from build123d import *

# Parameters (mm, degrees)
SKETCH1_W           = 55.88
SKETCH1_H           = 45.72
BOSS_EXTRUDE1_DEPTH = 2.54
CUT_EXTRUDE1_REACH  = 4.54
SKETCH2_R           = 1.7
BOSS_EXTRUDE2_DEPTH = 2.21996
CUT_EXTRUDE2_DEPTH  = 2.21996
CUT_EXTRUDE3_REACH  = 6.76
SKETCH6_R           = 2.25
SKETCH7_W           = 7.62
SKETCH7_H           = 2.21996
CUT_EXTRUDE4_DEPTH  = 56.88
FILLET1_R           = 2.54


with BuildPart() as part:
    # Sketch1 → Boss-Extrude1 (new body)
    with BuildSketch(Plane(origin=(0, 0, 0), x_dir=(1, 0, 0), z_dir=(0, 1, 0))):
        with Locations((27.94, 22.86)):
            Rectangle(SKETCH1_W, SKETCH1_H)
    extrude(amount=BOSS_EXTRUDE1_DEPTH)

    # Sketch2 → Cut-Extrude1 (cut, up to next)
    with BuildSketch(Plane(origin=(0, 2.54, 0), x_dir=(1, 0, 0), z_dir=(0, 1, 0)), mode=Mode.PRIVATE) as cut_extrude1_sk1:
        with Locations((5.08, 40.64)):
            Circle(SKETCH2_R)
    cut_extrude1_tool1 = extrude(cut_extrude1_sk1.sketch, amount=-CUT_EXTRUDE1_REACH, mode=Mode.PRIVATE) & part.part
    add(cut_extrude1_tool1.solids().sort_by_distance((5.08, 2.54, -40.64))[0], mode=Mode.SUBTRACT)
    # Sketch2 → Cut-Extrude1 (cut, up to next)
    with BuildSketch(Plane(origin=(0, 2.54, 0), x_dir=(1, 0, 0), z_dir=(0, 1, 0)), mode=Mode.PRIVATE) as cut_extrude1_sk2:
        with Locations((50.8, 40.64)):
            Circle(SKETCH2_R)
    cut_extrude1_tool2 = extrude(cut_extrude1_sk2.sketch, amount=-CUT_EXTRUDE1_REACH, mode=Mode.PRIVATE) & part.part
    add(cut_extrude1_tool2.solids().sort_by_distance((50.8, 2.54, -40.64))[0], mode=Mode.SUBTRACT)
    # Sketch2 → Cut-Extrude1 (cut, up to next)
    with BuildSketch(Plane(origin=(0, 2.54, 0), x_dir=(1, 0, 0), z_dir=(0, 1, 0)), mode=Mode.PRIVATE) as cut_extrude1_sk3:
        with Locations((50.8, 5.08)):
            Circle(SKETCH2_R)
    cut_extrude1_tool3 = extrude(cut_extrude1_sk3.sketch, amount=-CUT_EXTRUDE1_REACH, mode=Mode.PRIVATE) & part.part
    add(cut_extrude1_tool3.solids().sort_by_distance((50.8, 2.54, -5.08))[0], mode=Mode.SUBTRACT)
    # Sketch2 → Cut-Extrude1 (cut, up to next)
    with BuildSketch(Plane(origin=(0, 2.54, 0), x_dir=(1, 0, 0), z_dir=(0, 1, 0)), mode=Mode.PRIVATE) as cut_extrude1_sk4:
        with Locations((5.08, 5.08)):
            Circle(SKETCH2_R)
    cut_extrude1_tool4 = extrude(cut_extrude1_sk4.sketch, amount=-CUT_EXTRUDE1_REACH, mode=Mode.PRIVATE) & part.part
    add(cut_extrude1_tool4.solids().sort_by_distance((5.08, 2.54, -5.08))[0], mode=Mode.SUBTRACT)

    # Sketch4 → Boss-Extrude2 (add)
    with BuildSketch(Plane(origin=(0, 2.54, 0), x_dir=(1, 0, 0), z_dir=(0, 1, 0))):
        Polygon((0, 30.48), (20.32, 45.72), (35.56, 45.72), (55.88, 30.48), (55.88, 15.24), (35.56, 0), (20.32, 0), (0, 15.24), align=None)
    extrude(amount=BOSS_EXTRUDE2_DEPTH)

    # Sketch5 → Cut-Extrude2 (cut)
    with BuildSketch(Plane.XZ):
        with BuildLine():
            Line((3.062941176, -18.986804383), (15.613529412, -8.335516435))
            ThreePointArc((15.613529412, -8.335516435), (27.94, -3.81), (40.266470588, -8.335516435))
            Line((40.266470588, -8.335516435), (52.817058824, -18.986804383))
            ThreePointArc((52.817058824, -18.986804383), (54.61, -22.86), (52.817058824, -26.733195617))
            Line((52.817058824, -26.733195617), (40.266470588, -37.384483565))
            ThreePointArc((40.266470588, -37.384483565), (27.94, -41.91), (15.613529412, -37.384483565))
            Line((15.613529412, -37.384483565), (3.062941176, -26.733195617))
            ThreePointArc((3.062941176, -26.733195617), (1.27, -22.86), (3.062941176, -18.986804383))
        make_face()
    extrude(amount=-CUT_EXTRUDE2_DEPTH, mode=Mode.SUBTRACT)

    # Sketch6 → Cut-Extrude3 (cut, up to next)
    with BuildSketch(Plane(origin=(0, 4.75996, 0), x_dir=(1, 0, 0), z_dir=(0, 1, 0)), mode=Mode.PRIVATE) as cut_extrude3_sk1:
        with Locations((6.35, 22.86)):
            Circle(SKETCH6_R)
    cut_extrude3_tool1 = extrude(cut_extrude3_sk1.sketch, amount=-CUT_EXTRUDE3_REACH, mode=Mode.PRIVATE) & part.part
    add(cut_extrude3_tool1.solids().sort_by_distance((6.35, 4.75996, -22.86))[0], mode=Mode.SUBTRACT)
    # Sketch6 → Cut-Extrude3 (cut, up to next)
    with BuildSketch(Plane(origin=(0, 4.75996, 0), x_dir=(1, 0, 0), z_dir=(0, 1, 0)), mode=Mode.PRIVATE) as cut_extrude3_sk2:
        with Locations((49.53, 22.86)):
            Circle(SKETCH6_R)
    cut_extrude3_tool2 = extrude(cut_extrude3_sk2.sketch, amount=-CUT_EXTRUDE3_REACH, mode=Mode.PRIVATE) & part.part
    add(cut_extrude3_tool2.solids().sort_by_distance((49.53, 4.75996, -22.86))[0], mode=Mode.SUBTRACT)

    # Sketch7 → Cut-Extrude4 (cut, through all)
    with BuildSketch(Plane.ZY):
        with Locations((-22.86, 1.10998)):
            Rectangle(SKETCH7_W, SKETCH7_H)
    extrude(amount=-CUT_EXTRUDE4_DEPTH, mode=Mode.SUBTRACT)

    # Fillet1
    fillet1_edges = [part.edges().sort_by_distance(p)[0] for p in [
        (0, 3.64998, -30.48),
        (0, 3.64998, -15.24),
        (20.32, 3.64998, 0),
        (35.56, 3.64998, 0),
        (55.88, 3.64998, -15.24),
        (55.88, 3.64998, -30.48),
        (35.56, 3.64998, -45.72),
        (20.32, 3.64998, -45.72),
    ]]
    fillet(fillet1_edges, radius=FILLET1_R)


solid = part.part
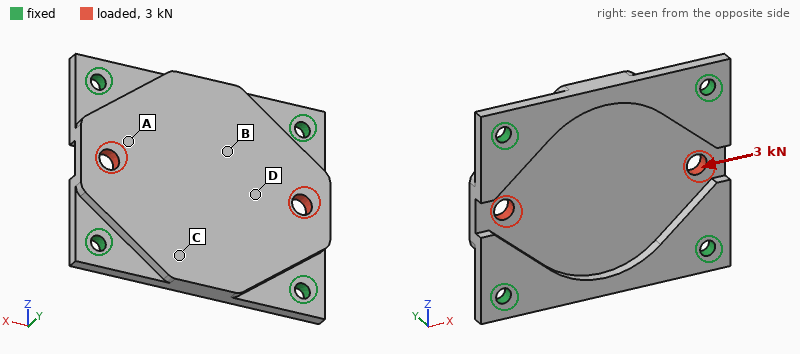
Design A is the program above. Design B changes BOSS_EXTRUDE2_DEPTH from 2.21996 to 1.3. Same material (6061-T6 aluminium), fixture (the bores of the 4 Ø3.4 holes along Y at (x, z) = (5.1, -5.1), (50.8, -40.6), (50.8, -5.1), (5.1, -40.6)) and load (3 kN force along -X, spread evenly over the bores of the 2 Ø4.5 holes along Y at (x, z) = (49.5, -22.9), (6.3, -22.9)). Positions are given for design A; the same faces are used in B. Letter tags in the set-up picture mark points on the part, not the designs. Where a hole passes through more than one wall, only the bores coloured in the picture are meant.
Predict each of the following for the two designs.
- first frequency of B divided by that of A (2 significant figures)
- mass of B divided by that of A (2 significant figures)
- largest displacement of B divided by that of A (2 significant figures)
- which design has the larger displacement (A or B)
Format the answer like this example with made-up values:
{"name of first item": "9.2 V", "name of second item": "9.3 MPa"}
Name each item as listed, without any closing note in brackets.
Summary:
{"first frequency of B divided by that of A": "0.87", "mass of B divided by that of A": "0.77", "largest displacement of B divided by that of A": "1.4", "which design has the larger displacement": "B"}
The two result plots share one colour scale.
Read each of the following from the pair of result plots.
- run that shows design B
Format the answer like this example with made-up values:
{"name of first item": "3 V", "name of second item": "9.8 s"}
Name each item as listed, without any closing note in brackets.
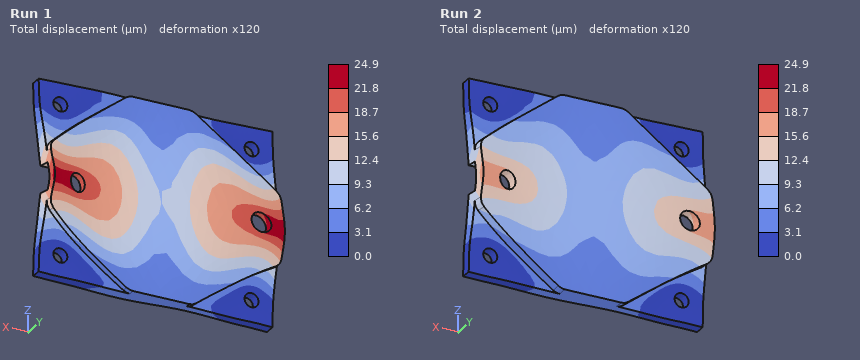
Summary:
{"run that shows design B": "Run 1"}
